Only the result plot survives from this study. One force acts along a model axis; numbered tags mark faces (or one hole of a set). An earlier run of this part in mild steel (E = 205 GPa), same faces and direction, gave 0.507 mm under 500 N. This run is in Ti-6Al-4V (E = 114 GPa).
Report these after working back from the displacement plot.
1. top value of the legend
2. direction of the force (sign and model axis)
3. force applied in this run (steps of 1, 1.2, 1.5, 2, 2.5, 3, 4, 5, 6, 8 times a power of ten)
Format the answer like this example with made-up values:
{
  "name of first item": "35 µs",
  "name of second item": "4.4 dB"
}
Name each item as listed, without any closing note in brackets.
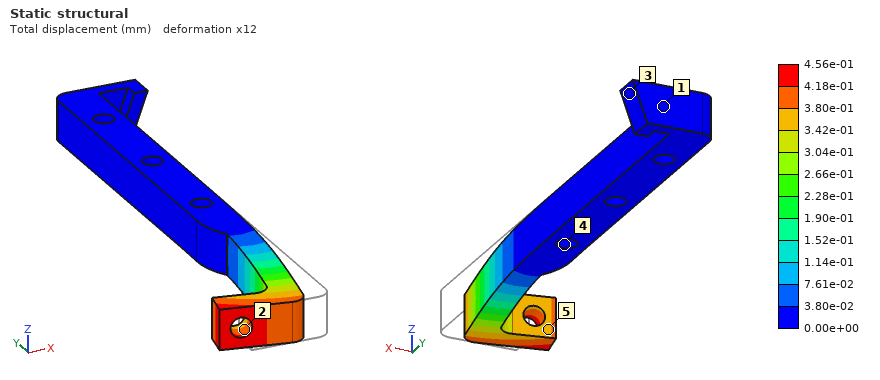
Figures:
{
  "top value of the legend": "4.56e-01 mm",
  "direction of the force": "-X",
  "force applied in this run": "250 N"
}
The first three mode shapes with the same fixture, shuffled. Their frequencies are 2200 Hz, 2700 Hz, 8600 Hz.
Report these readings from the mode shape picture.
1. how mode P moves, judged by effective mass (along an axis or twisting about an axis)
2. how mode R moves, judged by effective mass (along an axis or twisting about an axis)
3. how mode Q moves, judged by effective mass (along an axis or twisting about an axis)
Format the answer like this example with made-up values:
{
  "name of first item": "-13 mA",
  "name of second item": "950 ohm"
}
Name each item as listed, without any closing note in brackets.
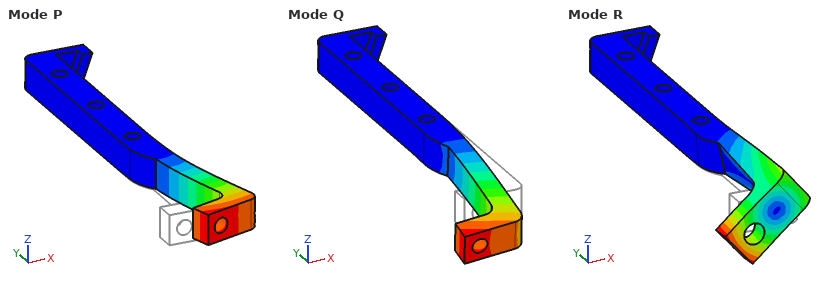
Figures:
{
  "how mode P moves, judged by effective mass": "along X",
  "how mode R moves, judged by effective mass": "twisting about Y",
  "how mode Q moves, judged by effective mass": "along Z"
}
